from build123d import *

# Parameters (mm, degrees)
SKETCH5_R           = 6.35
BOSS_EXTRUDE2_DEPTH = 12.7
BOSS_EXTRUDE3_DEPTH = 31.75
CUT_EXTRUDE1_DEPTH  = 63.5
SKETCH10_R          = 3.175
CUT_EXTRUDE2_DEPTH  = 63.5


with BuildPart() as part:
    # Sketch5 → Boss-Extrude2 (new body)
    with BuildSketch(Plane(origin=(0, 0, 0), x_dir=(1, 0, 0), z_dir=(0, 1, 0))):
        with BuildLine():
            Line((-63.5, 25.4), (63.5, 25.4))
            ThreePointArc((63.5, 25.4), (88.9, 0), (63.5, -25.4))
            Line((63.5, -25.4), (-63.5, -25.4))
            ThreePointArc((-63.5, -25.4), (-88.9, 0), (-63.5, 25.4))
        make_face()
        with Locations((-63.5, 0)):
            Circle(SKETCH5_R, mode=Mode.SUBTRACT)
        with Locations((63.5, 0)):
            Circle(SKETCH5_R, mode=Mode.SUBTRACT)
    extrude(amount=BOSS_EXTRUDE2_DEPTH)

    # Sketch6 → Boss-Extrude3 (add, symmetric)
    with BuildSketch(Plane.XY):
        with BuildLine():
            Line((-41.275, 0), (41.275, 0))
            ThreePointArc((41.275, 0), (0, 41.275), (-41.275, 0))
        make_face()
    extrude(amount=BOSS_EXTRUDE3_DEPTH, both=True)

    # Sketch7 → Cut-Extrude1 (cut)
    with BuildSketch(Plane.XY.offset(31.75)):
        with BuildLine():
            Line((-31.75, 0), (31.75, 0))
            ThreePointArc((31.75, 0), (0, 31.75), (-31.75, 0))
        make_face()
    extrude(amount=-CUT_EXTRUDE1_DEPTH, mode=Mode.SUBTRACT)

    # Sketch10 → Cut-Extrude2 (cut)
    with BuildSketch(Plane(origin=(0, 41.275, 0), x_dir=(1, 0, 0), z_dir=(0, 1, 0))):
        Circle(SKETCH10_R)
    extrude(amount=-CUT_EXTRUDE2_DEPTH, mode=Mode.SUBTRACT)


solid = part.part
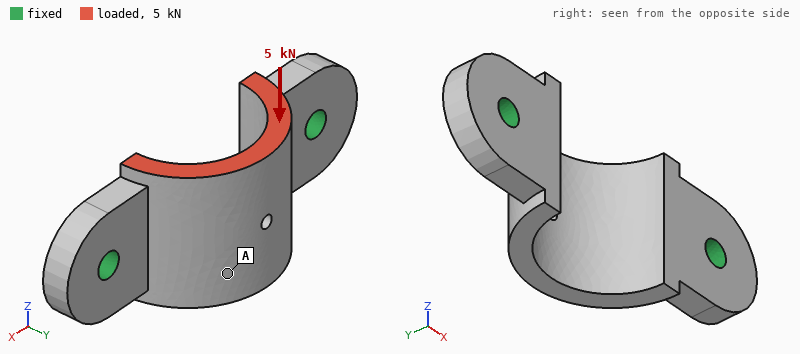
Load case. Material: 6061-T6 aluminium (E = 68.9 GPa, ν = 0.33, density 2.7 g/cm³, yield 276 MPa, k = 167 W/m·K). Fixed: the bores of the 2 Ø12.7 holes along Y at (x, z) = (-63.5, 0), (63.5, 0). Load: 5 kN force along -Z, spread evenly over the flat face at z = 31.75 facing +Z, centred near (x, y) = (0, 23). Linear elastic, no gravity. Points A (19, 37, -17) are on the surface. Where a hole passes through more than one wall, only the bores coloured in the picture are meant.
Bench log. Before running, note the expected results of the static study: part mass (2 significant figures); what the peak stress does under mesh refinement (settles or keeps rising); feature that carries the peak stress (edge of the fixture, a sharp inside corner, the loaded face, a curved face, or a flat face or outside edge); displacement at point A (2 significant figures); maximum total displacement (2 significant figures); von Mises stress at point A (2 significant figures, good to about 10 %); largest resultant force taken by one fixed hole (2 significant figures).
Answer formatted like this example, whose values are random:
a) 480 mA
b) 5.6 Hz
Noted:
a) 330 g
b) keeps rising
c) edge of the fixture
d) 69 µm
e) 93 µm
f) 7.3 MPa
g) 2.5 kN
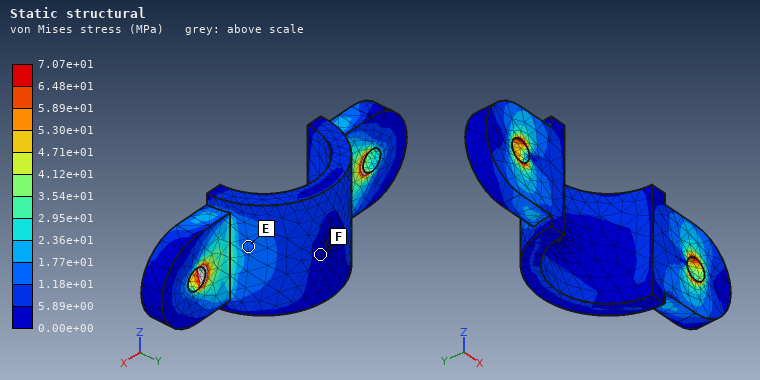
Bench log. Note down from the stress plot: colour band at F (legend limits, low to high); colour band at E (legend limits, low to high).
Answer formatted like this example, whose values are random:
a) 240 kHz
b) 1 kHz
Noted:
a) 0.00e+00 to 5.89e+00 MPa
b) 1.18e+01 to 1.77e+01 MPa
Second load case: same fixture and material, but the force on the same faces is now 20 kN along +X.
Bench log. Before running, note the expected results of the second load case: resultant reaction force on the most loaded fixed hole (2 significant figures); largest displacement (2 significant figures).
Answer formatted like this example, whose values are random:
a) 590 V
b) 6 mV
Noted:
a) 11 kN
b) 0.17 mm
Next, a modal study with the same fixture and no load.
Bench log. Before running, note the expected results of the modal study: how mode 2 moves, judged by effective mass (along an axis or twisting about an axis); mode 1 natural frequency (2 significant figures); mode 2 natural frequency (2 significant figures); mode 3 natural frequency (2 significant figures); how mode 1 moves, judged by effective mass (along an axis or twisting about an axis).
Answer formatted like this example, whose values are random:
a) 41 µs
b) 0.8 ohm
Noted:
a) along Y
b) 3000 Hz
c) 5700 Hz
d) 6300 Hz
e) along Z
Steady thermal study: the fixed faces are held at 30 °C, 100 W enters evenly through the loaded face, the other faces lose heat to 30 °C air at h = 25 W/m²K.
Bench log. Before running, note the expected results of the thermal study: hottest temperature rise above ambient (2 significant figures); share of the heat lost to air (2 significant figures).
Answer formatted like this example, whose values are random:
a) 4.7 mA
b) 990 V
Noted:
a) 33 K
b) 7.9 %
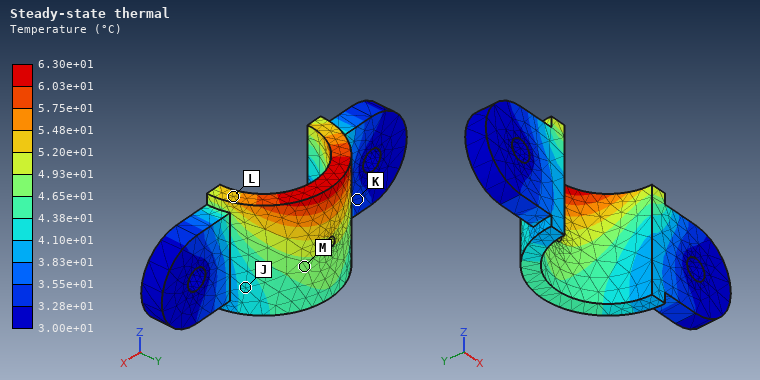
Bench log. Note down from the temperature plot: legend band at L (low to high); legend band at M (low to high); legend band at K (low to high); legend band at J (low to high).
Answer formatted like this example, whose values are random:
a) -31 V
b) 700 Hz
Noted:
a) 5.20e+01 to 5.48e+01 °C
b) 4.65e+01 to 4.93e+01 °C
c) 3.28e+01 to 3.55e+01 °C
d) 4.10e+01 to 4.38e+01 °C
